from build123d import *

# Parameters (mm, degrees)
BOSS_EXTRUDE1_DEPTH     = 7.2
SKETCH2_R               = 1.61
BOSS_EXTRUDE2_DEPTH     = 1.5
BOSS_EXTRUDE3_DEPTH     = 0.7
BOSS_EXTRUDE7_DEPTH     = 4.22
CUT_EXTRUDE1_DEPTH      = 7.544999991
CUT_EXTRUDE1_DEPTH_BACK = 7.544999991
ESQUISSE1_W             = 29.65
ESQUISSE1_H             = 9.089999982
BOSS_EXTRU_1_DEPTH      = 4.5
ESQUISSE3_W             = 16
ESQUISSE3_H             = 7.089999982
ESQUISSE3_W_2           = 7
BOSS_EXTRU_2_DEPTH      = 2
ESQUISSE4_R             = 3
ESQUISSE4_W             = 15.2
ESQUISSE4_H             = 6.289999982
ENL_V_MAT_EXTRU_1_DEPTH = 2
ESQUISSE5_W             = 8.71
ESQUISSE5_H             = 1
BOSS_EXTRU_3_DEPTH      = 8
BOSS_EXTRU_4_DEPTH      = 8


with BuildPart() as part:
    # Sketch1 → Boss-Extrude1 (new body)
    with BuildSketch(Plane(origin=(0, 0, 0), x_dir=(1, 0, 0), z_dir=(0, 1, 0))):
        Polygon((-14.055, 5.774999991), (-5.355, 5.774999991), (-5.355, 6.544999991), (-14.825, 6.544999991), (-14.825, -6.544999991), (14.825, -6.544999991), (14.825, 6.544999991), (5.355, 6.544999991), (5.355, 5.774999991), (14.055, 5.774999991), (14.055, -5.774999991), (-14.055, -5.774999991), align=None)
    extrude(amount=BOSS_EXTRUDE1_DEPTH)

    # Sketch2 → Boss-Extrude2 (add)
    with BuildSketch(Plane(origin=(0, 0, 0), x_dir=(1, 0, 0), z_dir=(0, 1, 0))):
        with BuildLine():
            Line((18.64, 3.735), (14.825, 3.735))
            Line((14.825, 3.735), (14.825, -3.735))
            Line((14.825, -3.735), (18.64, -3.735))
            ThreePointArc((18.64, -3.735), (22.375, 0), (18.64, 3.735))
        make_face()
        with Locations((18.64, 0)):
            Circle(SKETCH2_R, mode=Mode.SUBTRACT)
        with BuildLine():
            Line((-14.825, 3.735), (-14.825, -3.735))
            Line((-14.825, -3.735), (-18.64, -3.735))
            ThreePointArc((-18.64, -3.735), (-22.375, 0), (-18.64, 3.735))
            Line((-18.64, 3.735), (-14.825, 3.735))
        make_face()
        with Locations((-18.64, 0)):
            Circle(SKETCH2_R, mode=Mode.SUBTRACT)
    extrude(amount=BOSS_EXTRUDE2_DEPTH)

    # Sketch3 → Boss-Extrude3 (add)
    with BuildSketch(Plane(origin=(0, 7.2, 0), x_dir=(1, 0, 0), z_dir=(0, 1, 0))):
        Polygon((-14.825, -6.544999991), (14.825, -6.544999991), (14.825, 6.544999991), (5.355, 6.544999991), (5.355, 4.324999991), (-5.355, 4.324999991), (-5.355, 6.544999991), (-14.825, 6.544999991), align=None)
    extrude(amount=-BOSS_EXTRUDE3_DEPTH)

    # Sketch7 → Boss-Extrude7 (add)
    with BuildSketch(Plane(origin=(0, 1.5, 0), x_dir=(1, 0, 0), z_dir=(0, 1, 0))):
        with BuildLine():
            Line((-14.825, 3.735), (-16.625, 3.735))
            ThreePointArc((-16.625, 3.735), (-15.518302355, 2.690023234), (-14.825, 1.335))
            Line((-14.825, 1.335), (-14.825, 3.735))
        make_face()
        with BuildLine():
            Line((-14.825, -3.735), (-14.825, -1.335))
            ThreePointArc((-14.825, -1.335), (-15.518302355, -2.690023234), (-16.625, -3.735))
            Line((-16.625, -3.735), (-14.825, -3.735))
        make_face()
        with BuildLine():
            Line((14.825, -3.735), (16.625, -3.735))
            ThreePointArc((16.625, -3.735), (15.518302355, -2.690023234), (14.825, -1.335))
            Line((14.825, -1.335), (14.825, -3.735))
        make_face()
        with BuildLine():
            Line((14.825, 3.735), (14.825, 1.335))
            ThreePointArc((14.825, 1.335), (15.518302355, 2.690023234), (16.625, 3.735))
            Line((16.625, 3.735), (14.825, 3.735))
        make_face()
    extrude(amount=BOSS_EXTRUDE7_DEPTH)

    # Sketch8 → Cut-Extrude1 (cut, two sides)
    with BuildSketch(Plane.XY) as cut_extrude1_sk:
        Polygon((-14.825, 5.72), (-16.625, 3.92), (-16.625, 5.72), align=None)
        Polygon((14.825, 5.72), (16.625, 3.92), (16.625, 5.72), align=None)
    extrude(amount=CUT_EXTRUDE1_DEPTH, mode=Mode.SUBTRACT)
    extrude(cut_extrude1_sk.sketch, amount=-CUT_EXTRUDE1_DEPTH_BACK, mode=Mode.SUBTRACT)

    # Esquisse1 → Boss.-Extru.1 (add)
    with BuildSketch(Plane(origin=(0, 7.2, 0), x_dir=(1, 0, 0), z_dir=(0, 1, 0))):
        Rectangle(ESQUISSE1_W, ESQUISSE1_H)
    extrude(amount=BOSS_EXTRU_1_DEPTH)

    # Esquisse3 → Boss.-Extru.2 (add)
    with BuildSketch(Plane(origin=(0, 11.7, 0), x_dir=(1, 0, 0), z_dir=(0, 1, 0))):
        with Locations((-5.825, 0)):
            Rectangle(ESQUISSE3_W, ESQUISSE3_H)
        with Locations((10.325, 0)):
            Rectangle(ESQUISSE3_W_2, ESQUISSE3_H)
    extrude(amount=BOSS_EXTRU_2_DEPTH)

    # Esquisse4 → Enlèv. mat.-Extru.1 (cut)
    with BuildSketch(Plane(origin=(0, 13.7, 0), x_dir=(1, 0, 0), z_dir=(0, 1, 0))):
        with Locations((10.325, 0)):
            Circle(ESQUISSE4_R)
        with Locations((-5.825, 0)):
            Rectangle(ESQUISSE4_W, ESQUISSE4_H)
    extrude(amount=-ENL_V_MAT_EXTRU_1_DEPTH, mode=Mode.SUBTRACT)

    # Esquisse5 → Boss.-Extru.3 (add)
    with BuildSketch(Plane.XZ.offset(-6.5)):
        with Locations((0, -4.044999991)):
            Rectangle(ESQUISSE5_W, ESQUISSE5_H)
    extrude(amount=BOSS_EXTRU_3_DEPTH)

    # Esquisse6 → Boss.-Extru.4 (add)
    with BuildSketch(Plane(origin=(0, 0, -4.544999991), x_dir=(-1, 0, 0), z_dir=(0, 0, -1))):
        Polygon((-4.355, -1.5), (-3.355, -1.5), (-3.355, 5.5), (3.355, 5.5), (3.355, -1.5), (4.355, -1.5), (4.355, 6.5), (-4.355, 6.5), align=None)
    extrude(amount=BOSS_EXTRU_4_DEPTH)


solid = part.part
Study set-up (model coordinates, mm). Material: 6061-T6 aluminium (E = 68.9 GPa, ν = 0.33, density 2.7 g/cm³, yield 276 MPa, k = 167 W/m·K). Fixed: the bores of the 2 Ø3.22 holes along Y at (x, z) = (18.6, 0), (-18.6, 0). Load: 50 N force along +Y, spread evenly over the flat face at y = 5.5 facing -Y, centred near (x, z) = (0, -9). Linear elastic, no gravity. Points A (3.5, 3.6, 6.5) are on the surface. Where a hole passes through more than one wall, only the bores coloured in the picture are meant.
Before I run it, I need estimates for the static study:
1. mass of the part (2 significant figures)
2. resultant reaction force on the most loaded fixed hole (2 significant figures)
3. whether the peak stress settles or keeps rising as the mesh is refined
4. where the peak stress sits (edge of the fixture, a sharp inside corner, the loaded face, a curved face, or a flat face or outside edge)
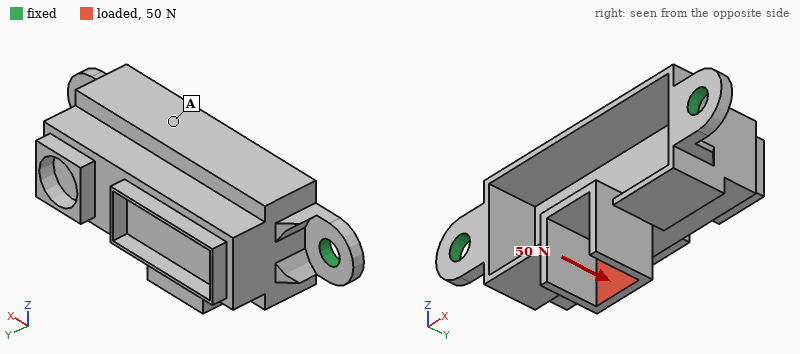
6.2 g
28 N
keeps rising
a sharp inside corner
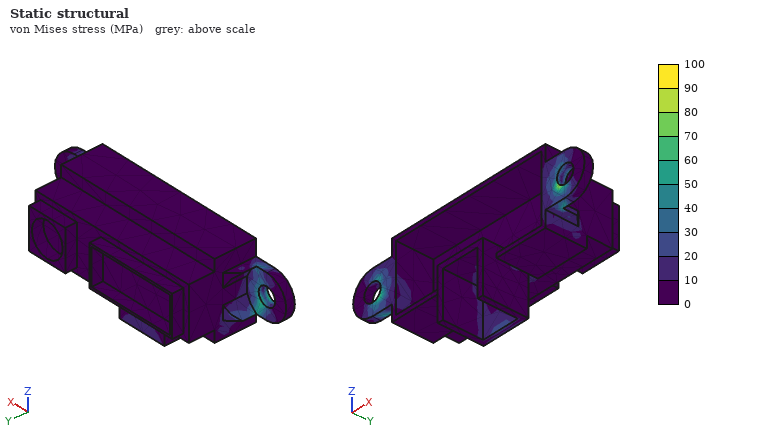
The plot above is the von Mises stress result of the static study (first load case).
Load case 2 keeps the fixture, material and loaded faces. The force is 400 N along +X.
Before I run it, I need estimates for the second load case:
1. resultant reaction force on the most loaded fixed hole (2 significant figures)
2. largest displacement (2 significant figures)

230 N
91 µm
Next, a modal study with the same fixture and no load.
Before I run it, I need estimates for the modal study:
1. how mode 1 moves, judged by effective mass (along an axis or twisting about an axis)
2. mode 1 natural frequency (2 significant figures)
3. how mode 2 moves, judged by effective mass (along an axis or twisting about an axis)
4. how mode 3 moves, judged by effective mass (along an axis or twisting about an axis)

along Z
3900 Hz
along Z
along X
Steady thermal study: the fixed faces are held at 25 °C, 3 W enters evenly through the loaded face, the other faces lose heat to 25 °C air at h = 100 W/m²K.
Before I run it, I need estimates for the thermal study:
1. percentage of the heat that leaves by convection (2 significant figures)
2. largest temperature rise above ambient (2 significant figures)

45 %
13 K
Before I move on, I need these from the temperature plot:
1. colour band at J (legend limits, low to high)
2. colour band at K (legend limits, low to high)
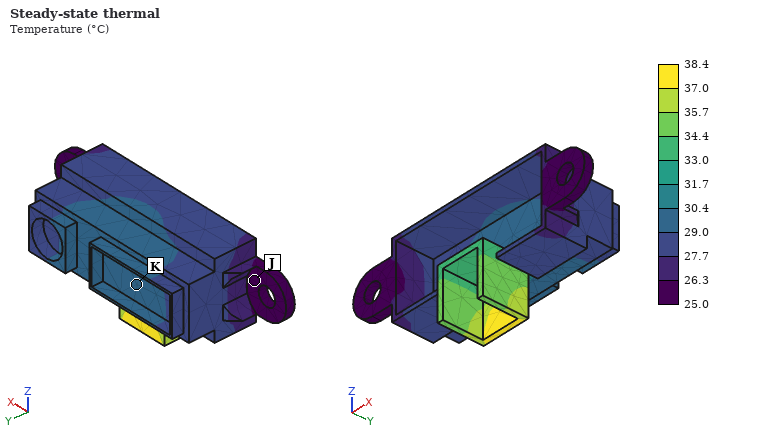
25.0 to 26.3 °C
29.0 to 30.4 °C
